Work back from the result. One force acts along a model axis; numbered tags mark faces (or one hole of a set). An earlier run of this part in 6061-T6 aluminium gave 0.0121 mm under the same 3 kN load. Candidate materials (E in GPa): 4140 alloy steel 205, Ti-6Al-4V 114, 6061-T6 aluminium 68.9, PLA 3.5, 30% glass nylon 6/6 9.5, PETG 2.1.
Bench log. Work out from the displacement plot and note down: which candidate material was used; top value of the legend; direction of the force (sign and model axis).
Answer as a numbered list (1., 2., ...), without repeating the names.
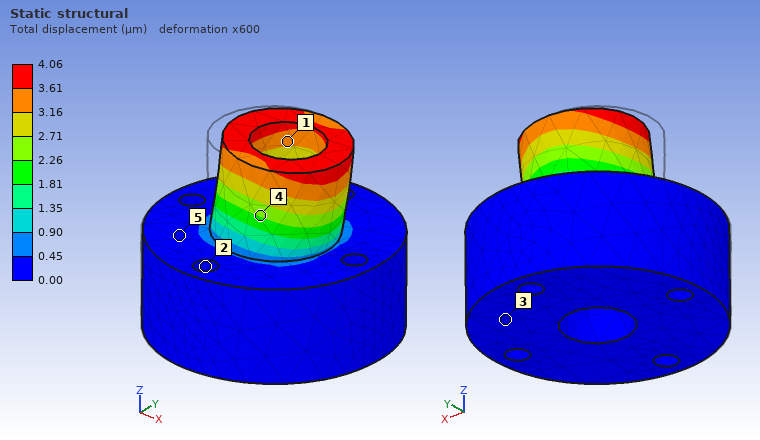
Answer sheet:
1. 4140 alloy steel
2. 4.06 µm
3. +X
